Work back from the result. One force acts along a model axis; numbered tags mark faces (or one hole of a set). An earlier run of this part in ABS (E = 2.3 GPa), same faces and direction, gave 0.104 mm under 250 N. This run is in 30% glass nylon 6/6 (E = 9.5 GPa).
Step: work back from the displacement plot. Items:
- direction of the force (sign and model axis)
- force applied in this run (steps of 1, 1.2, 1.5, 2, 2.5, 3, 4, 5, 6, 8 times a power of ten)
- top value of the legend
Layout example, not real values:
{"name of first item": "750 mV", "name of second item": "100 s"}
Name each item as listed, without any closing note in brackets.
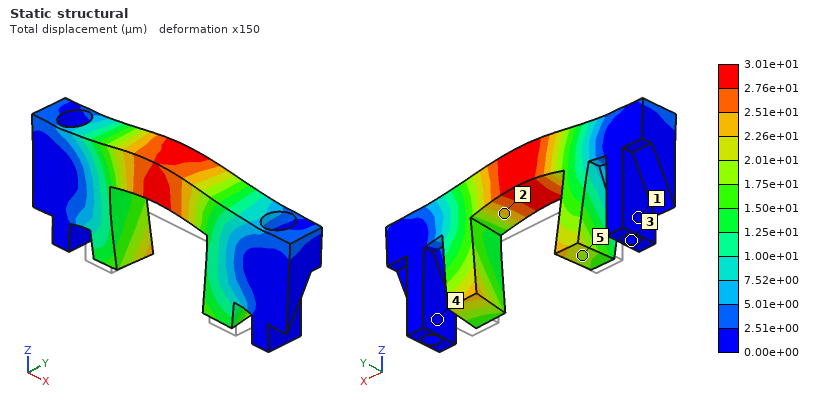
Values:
{"direction of the force": "+Z", "force applied in this run": "300 N", "top value of the legend": "3.01e+01 µm"}
